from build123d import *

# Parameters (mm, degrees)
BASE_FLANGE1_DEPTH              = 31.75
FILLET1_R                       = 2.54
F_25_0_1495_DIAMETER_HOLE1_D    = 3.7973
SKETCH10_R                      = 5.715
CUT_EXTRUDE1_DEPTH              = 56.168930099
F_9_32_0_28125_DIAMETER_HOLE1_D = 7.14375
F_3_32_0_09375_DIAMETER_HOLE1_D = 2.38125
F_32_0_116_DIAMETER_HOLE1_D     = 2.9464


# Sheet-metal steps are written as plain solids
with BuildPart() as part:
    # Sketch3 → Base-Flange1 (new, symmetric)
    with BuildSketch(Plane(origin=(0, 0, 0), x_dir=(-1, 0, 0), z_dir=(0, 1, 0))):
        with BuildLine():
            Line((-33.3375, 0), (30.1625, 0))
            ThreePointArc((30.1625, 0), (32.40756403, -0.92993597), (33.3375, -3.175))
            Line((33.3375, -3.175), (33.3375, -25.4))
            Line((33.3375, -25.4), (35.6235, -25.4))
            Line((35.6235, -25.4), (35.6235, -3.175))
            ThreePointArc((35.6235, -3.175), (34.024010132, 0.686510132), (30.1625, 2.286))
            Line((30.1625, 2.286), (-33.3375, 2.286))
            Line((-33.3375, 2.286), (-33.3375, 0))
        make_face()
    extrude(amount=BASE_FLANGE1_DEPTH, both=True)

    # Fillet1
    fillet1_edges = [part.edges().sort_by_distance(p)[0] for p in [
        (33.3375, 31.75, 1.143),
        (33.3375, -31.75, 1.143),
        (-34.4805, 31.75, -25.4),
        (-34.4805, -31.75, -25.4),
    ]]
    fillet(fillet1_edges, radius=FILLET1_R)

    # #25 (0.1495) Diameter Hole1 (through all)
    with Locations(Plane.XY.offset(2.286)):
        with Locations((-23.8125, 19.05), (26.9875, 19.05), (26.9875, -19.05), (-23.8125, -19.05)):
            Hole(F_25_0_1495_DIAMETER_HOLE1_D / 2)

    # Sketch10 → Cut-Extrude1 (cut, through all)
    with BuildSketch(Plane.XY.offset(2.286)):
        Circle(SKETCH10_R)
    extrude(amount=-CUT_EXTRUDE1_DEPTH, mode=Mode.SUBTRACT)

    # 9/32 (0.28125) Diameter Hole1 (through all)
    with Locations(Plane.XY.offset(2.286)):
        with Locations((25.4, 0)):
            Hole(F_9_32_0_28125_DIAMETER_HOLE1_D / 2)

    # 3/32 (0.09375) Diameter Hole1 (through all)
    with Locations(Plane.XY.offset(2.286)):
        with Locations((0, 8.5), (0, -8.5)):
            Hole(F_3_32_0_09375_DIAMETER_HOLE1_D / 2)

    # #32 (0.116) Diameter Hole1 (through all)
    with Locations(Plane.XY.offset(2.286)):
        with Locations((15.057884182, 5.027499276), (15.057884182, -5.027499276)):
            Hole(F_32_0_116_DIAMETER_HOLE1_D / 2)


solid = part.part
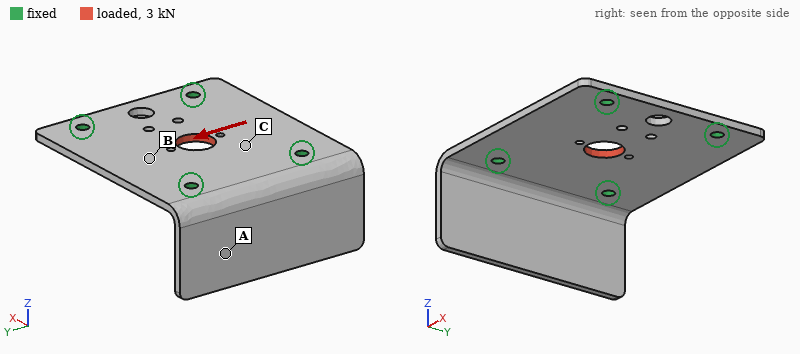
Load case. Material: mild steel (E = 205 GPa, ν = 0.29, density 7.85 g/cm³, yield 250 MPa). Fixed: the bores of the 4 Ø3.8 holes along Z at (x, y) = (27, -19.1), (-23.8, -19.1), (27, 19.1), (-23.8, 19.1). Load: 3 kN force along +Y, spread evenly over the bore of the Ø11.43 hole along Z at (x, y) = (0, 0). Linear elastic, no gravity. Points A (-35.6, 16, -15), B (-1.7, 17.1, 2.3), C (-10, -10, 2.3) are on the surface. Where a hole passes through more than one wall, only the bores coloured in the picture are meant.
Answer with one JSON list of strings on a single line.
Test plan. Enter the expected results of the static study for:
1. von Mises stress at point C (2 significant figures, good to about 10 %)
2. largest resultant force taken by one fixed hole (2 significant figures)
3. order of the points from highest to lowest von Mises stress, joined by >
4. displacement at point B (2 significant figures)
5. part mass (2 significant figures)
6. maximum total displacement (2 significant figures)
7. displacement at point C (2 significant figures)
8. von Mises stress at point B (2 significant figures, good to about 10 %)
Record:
["27 MPa", "890 N", "C > B > A", "3.7 µm", "100 g", "5.6 µm", "3.0 µm", "13 MPa"]
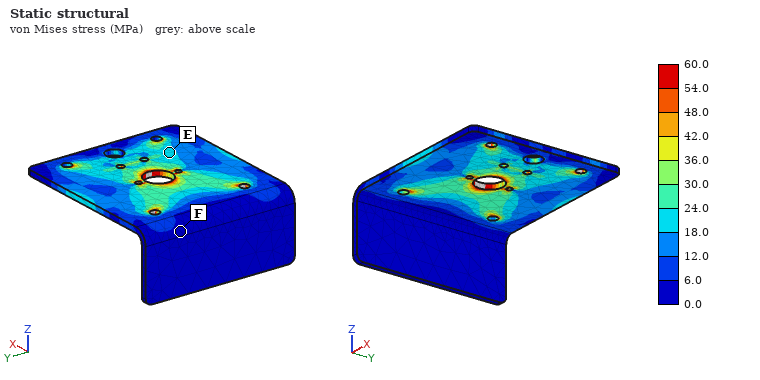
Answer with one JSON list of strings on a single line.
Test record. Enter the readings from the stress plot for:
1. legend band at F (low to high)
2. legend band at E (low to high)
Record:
["0.0 to 6.0 MPa", "18.0 to 24.0 MPa"]
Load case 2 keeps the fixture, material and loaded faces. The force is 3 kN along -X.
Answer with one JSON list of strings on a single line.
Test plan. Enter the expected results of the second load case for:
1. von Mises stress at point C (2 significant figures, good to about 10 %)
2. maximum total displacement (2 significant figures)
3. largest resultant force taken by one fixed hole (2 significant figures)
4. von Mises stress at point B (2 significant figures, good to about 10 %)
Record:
["23 MPa", "4.2 µm", "850 N", "10 MPa"]
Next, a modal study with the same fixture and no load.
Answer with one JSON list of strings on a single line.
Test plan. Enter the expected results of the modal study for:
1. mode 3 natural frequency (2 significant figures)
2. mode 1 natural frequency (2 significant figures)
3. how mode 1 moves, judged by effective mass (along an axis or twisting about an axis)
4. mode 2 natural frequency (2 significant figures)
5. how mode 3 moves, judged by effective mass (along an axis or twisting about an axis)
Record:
["4100 Hz", "1700 Hz", "along X", "2800 Hz", "along Z"]
